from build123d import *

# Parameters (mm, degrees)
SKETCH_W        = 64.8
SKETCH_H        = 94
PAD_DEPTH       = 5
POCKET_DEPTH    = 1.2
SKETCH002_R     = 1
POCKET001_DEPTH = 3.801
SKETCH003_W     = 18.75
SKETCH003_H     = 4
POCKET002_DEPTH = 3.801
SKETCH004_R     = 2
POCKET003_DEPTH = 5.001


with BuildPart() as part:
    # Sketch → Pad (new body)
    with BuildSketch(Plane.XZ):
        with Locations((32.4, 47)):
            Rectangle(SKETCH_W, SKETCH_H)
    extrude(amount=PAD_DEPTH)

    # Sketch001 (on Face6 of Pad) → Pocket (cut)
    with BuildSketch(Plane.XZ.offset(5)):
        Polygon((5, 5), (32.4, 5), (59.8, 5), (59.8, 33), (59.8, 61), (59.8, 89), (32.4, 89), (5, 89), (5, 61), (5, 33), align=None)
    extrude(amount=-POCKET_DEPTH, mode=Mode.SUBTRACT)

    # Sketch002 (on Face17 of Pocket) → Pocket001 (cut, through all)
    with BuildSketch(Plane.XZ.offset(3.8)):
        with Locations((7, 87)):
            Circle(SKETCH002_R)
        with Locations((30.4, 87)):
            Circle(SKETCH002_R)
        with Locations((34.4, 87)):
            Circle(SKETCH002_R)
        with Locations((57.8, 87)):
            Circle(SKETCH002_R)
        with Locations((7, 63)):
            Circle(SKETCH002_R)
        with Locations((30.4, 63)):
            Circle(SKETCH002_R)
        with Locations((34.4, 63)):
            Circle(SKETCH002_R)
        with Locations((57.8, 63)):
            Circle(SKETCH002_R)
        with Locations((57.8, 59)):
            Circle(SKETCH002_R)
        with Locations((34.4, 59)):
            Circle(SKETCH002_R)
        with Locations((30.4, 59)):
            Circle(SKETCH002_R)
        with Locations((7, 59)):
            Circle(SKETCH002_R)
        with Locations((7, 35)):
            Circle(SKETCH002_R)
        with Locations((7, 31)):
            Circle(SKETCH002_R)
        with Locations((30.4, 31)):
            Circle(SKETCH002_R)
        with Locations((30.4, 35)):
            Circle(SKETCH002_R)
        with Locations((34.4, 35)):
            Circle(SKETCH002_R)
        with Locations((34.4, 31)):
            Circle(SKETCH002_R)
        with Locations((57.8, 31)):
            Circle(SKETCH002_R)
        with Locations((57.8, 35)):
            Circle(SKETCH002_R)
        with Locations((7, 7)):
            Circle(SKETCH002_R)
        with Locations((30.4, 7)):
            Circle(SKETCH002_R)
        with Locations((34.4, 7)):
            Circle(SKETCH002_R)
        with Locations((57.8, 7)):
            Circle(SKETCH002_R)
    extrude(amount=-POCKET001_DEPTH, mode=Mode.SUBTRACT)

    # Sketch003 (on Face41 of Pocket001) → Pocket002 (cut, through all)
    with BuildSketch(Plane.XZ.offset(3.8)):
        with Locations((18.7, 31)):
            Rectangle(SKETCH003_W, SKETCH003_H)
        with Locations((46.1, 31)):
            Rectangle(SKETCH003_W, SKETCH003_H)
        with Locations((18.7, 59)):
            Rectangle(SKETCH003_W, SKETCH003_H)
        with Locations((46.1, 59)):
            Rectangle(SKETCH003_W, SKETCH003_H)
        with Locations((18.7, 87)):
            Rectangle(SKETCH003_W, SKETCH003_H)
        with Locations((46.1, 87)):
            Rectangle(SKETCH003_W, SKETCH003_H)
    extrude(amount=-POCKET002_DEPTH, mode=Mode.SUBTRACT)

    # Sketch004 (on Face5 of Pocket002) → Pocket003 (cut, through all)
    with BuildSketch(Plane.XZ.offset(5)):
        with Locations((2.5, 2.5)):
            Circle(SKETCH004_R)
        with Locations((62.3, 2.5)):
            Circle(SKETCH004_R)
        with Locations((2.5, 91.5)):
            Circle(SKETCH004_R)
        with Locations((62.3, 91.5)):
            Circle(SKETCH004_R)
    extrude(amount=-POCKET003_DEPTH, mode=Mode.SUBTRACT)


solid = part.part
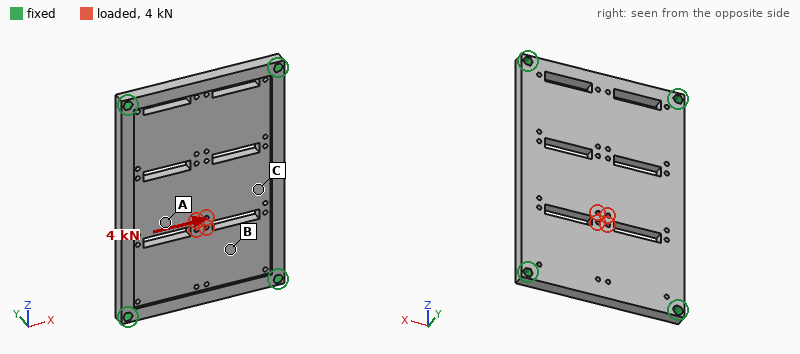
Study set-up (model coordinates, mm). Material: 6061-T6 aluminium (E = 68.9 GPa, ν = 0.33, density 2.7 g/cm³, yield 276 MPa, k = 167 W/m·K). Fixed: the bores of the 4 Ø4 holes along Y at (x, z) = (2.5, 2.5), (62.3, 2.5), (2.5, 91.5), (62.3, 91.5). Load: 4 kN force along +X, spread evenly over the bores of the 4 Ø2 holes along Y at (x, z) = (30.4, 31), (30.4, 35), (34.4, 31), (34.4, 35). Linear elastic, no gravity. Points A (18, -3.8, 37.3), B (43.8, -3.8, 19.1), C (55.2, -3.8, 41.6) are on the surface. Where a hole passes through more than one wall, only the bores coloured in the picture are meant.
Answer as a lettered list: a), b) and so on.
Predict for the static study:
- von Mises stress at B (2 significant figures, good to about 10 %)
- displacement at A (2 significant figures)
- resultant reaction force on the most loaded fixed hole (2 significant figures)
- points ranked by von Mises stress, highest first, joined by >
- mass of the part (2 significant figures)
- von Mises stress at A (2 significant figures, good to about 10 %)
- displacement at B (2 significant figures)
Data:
a) 32 MPa
b) 29 µm
c) 1.6 kN
d) B > A > C
e) 61 g
f) 21 MPa
g) 13 µm
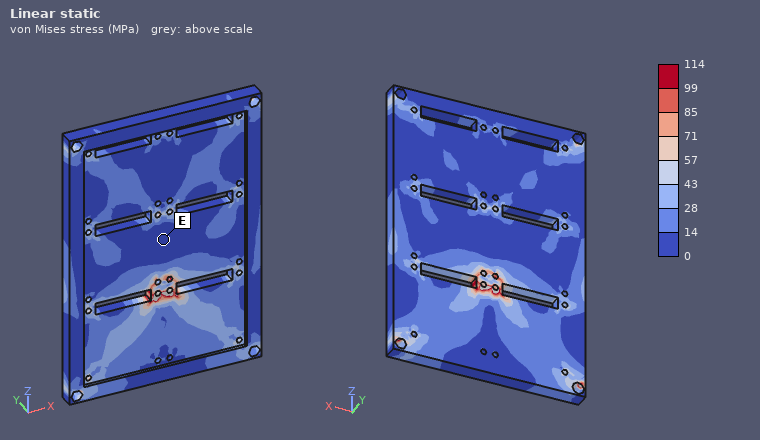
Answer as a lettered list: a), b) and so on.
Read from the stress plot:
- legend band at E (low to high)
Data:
a) 0 to 14 MPa
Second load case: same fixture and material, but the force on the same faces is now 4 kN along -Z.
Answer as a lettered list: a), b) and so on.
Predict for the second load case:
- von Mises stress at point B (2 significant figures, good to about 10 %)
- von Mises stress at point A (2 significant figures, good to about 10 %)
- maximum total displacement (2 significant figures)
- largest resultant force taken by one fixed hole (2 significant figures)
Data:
a) 25 MPa
b) 9.7 MPa
c) 25 µm
d) 1.4 kN
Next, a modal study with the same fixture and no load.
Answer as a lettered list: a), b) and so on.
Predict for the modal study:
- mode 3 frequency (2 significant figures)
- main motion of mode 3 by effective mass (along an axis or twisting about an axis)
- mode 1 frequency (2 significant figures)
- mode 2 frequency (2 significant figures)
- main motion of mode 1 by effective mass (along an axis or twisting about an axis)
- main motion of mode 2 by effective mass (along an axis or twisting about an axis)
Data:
a) 4700 Hz
b) twisting about X
c) 2000 Hz
d) 3500 Hz
e) along Y
f) twisting about Z
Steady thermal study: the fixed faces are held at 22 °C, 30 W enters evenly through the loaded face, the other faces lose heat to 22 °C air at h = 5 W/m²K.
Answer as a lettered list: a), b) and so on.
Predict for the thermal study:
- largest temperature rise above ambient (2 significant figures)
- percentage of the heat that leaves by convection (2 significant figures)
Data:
a) 38 K
b) 3.2 %
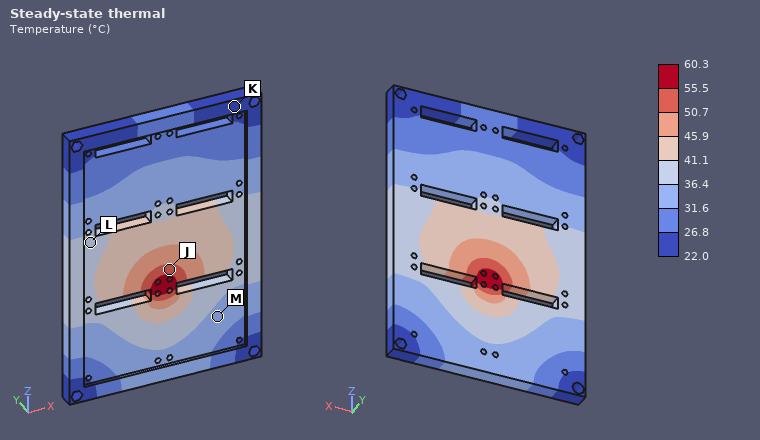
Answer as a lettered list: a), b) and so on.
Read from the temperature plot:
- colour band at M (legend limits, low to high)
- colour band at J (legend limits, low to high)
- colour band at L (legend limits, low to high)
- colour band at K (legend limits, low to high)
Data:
a) 31.6 to 36.4 °C
b) 50.7 to 55.5 °C
c) 36.4 to 41.1 °C
d) 22.0 to 26.8 °C
